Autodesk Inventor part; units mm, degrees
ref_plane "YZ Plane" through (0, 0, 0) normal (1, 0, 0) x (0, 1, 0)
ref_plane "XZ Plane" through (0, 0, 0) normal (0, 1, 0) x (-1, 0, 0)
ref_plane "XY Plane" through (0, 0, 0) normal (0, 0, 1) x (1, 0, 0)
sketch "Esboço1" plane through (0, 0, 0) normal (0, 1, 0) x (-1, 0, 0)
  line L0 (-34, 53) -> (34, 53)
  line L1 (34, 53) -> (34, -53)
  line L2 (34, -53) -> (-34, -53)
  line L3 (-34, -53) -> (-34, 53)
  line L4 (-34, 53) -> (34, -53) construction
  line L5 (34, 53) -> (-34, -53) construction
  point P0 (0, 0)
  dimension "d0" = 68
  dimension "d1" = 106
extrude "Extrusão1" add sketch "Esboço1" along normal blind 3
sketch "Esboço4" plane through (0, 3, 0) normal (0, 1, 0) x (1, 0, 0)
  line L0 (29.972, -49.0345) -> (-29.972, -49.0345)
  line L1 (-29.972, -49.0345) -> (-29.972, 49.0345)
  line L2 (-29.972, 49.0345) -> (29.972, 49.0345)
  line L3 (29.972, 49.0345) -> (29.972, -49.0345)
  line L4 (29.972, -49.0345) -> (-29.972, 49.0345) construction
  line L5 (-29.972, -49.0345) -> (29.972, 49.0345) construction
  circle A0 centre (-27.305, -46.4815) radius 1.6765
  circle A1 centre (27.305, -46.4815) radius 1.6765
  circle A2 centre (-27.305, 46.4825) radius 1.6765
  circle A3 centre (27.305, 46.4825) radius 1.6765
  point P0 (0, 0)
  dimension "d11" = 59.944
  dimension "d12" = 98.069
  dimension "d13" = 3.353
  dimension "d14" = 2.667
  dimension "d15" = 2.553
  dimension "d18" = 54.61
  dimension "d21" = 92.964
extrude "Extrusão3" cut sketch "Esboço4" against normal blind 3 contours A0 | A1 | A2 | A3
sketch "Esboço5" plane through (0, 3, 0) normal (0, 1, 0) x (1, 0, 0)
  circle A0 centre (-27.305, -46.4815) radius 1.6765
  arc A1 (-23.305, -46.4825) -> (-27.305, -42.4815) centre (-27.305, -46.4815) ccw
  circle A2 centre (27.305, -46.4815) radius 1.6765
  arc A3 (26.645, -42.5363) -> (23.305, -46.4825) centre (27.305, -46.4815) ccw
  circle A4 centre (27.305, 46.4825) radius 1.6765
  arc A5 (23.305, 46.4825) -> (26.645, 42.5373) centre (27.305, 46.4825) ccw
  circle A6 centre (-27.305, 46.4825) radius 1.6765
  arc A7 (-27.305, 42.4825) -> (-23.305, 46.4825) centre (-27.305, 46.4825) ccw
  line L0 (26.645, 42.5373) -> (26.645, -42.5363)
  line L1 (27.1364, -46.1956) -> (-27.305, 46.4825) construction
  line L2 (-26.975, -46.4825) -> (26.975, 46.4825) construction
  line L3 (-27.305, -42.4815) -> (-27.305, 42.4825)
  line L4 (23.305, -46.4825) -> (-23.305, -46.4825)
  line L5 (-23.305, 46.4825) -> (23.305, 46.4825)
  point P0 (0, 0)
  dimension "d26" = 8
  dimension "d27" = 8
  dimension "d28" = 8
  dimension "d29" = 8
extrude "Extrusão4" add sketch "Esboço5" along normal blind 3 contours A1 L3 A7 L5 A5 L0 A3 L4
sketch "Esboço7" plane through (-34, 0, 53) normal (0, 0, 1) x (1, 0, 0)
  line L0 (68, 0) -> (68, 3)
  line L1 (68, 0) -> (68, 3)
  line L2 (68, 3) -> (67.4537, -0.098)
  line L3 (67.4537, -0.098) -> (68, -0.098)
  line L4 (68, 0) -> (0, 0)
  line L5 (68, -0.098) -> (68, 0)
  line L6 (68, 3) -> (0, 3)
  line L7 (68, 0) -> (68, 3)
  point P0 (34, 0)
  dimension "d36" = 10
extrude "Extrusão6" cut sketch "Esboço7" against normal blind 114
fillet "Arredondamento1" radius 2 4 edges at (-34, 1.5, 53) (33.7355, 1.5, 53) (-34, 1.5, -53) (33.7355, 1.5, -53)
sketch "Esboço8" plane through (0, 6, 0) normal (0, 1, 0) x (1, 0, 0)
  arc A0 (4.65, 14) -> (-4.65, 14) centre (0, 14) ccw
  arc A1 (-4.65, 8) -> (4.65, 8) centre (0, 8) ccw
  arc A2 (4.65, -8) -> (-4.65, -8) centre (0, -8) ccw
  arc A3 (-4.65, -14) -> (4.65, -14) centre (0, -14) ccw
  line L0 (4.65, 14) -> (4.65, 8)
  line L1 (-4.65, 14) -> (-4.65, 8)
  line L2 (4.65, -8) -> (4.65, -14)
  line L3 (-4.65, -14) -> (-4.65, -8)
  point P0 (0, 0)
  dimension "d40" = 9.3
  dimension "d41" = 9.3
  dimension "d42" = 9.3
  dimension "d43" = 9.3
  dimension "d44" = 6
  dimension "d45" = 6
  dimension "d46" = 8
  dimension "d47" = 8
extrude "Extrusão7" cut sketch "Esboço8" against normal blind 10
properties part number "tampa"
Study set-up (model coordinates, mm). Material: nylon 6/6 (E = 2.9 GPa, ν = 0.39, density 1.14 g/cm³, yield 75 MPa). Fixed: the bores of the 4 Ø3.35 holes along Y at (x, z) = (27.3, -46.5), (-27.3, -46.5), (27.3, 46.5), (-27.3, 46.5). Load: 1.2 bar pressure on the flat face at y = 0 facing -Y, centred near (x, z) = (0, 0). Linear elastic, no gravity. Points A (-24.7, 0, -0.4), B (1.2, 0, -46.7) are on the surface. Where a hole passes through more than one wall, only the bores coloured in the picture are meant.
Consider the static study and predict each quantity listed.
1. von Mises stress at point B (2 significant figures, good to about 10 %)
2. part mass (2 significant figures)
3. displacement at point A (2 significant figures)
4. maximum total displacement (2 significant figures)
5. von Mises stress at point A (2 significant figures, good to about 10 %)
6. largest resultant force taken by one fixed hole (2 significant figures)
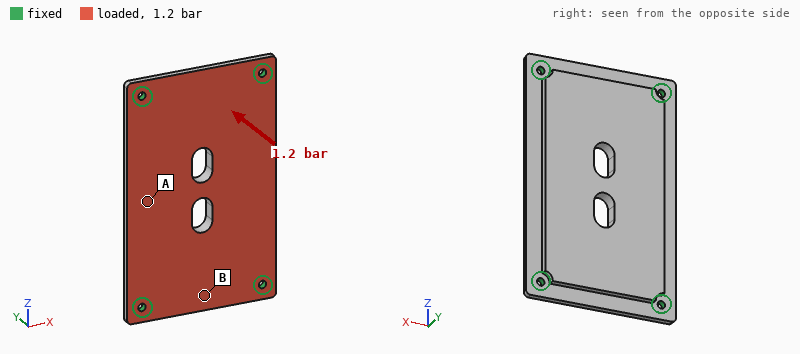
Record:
5.7 MPa
40 g
1.4 mm
1.5 mm
13 MPa
400 N
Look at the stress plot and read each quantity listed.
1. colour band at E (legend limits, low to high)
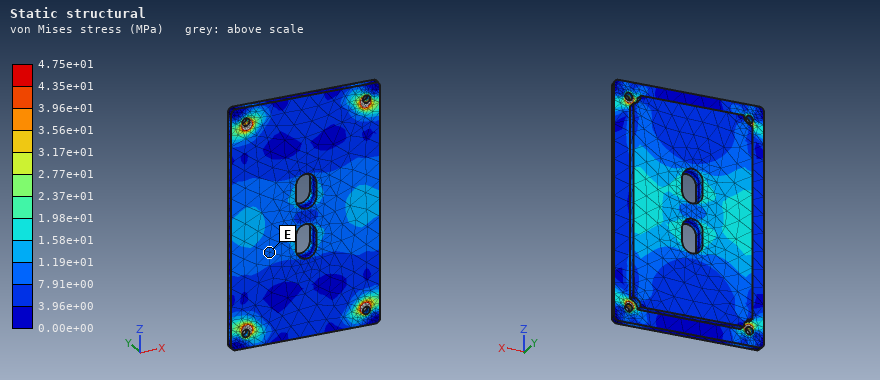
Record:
7.91e+00 to 1.19e+01 MPa
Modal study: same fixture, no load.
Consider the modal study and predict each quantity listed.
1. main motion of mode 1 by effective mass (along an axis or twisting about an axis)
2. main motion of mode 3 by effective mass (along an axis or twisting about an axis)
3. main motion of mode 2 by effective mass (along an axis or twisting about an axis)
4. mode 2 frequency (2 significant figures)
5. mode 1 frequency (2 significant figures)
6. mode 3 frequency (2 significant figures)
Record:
along Y
twisting about X
twisting about Z
1200 Hz
680 Hz
1800 Hz
